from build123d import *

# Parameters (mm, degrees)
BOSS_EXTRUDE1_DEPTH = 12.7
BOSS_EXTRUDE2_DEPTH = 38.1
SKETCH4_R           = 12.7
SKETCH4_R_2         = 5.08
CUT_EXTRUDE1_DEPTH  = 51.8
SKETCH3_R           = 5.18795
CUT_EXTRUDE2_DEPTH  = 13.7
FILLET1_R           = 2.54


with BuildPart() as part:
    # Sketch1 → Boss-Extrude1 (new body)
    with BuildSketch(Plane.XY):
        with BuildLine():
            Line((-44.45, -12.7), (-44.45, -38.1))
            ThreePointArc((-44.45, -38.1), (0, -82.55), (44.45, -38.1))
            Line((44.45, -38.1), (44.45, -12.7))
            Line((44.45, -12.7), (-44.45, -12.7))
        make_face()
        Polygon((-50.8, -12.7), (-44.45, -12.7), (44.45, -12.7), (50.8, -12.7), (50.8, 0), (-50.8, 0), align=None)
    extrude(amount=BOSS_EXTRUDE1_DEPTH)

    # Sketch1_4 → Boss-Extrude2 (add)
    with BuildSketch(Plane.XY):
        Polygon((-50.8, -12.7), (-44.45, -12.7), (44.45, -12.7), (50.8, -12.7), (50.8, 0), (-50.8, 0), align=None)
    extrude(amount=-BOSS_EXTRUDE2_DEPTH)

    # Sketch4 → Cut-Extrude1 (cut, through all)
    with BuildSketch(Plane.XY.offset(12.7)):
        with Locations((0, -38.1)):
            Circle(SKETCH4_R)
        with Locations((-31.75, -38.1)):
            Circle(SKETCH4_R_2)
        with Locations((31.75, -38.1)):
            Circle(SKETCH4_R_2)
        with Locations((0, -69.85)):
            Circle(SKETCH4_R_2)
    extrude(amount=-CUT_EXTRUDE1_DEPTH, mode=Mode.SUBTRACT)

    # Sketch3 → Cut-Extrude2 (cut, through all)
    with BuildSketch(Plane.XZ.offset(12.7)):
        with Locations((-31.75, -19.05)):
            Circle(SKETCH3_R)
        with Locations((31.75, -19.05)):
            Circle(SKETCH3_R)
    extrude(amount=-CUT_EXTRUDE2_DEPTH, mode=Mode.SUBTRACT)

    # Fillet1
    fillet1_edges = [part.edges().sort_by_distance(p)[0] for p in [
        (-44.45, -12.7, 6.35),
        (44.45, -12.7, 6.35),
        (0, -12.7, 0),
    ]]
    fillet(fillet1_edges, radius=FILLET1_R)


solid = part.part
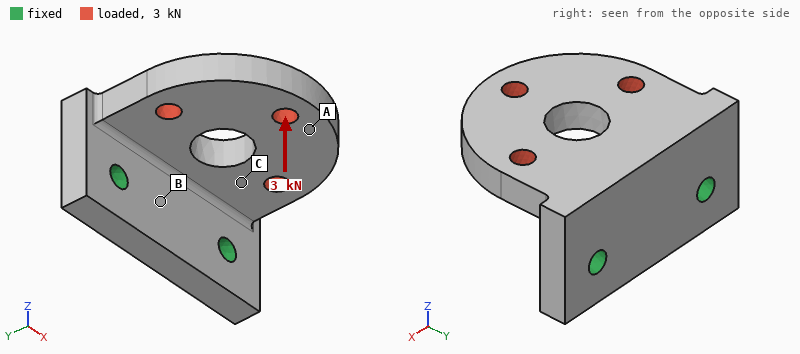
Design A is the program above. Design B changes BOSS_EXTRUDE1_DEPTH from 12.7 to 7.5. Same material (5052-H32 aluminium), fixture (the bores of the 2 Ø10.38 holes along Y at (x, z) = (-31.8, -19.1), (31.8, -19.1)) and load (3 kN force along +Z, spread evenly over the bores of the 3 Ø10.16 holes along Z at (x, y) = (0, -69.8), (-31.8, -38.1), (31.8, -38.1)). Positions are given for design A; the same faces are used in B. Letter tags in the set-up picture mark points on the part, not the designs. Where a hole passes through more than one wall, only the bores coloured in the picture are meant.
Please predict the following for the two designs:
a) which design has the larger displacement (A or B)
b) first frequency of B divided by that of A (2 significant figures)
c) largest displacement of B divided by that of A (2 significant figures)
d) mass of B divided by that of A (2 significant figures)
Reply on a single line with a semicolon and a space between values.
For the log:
B; 0.82; 2.7; 0.75
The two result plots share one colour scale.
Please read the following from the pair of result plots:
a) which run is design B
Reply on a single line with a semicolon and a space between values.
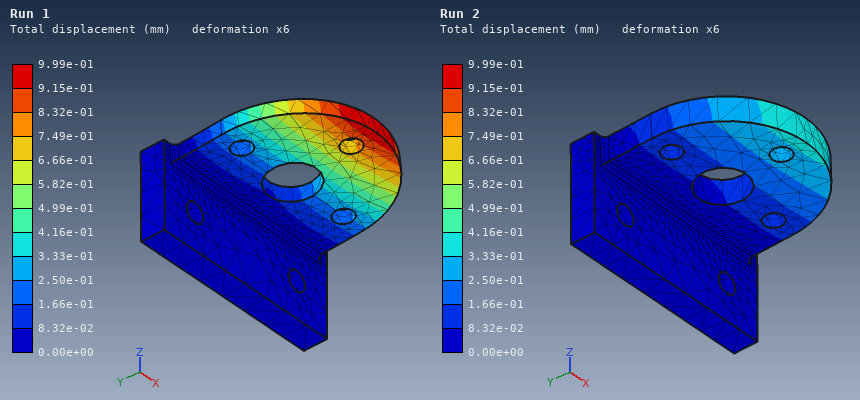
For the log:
Run 1
